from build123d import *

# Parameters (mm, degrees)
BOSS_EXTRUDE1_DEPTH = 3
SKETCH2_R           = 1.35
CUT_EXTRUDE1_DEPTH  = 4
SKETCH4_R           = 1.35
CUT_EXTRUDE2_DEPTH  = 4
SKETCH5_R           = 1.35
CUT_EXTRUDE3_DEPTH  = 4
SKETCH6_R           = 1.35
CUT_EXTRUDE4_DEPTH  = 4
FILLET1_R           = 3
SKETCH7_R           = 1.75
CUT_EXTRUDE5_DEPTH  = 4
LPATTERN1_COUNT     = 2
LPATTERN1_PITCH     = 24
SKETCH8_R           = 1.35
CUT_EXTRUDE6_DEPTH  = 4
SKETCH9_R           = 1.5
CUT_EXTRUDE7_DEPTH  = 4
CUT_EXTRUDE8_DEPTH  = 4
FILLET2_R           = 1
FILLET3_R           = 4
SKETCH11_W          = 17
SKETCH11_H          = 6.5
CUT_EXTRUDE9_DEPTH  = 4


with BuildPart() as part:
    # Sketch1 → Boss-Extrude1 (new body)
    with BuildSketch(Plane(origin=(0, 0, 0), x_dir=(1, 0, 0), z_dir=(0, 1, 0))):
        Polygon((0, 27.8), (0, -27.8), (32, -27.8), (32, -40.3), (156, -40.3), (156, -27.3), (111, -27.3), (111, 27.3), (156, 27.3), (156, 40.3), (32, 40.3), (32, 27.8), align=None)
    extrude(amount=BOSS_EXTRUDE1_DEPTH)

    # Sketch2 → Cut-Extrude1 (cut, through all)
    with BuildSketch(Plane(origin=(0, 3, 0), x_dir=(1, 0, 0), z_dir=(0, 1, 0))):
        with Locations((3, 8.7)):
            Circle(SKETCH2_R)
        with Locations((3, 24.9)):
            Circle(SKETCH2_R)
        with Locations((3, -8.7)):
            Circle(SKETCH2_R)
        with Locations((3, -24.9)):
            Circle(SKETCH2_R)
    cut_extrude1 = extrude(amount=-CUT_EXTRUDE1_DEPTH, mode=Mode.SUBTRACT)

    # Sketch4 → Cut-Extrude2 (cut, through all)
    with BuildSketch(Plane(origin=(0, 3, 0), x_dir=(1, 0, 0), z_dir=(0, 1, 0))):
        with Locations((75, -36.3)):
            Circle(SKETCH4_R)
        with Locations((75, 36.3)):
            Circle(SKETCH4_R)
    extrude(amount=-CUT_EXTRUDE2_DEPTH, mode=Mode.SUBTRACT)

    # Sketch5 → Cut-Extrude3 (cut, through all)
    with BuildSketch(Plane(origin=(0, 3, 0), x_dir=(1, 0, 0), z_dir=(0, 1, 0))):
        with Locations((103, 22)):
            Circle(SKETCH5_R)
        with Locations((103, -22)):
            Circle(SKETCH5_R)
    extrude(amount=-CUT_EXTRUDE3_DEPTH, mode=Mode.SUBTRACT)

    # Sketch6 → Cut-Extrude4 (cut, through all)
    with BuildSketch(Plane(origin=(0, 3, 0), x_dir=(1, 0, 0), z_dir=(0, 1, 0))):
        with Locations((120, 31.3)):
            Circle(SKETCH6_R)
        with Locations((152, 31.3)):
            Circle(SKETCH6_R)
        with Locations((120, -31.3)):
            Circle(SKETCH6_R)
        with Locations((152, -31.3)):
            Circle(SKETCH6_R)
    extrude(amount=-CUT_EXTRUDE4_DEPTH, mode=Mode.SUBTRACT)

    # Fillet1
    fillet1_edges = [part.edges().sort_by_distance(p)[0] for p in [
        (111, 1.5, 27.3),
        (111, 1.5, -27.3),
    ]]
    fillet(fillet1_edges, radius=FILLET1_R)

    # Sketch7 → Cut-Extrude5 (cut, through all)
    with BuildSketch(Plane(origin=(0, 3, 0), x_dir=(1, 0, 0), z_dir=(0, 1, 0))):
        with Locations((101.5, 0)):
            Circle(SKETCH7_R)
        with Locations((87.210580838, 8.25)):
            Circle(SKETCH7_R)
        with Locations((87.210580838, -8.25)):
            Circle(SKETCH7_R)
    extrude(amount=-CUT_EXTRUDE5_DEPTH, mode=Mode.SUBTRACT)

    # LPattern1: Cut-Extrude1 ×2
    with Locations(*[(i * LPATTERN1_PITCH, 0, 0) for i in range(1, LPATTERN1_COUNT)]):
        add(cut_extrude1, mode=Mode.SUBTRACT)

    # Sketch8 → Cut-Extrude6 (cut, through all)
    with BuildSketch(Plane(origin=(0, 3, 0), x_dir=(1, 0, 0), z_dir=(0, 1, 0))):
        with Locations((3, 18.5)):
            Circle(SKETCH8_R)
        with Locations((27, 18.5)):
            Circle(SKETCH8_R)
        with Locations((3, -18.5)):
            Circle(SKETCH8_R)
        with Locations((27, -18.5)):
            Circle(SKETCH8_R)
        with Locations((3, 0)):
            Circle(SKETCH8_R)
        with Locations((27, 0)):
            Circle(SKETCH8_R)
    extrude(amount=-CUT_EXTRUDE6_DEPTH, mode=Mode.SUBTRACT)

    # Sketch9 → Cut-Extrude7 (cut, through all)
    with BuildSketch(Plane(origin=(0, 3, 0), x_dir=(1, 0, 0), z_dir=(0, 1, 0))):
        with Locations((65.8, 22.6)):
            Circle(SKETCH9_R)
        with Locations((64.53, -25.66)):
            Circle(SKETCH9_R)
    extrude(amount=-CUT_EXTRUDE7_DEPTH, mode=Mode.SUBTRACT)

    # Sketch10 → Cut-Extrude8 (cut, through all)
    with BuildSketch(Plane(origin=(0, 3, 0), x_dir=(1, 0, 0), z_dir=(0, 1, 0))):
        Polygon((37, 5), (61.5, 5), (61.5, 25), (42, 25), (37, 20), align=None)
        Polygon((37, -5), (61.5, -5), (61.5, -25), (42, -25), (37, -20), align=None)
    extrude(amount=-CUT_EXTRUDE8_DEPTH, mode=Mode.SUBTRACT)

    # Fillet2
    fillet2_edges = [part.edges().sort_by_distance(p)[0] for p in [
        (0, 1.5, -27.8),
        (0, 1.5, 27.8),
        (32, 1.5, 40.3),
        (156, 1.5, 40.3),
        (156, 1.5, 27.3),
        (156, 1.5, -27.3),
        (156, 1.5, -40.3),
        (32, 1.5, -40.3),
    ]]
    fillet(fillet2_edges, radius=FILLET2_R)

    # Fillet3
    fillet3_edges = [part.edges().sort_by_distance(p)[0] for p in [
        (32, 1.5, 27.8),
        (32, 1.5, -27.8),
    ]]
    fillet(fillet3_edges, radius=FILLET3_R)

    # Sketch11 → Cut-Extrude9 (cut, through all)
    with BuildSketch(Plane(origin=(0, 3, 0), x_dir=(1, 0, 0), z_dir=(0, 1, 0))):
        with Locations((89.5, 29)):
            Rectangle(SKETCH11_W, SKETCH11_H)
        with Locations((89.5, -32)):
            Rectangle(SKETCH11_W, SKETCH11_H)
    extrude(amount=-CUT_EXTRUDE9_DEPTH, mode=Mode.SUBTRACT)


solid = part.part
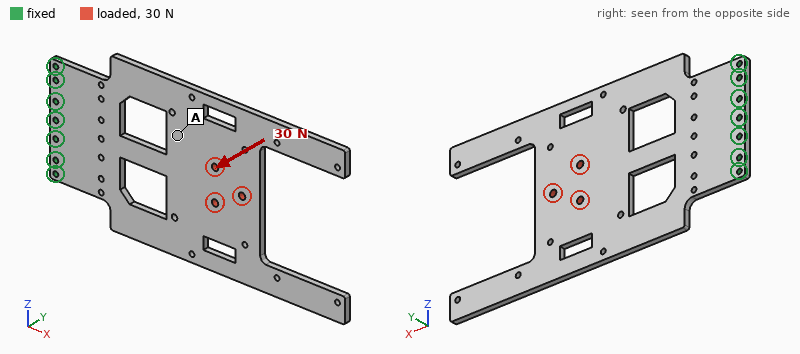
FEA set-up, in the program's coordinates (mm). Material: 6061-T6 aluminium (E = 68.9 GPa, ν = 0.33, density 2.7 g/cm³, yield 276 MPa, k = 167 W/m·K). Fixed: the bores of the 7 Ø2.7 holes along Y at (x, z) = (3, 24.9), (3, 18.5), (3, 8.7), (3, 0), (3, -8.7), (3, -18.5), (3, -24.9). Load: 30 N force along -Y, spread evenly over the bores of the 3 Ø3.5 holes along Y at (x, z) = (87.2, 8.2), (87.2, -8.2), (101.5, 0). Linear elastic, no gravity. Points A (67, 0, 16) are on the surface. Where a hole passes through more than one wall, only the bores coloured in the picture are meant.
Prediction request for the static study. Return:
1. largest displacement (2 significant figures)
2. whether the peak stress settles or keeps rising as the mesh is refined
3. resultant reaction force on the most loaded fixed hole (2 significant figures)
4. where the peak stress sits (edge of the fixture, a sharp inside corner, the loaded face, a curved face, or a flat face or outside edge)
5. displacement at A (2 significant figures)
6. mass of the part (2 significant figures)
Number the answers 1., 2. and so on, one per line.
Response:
1. 2.0 mm
2. keeps rising
3. 19 N
4. edge of the fixture
5. 0.54 mm
6. 65 g
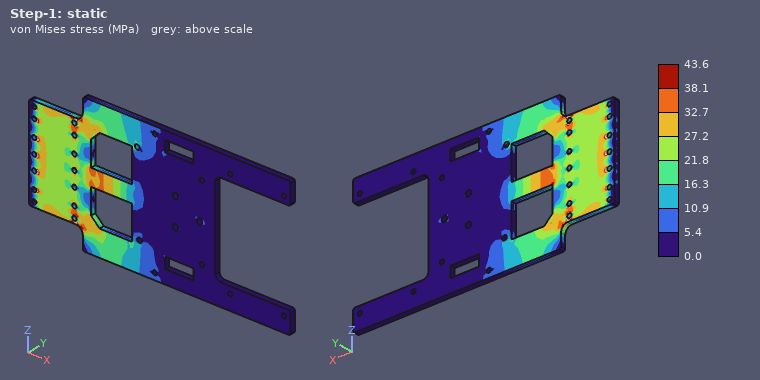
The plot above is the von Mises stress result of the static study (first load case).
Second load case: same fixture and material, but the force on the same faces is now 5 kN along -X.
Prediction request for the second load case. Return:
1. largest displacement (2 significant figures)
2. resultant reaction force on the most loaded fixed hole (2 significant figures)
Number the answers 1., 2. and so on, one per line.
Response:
1. 76 µm
2. 750 N
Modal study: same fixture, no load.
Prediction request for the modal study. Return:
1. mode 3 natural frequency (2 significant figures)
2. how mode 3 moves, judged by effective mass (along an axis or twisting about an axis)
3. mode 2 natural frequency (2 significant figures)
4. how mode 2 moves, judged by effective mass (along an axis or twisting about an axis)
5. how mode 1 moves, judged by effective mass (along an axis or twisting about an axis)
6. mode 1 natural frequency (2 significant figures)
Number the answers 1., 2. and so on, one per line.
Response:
1. 670 Hz
2. along Y
3. 340 Hz
4. twisting about X
5. along Y
6. 120 Hz
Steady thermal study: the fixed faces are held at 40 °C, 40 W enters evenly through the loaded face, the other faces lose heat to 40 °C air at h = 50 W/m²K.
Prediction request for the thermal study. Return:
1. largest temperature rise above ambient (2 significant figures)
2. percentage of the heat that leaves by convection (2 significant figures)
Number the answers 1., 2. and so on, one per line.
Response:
1. 65 K
2. 74 %
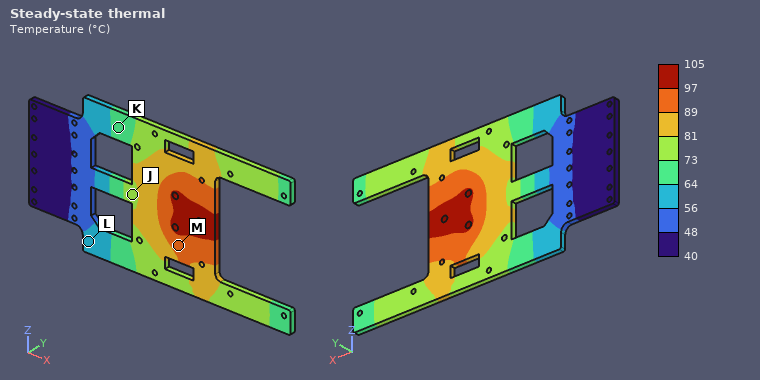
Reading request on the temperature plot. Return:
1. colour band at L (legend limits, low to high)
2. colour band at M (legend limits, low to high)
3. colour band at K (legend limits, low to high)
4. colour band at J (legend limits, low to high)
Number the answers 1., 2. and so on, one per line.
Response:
1. 56 to 64 °C
2. 89 to 97 °C
3. 64 to 73 °C
4. 73 to 81 °C
